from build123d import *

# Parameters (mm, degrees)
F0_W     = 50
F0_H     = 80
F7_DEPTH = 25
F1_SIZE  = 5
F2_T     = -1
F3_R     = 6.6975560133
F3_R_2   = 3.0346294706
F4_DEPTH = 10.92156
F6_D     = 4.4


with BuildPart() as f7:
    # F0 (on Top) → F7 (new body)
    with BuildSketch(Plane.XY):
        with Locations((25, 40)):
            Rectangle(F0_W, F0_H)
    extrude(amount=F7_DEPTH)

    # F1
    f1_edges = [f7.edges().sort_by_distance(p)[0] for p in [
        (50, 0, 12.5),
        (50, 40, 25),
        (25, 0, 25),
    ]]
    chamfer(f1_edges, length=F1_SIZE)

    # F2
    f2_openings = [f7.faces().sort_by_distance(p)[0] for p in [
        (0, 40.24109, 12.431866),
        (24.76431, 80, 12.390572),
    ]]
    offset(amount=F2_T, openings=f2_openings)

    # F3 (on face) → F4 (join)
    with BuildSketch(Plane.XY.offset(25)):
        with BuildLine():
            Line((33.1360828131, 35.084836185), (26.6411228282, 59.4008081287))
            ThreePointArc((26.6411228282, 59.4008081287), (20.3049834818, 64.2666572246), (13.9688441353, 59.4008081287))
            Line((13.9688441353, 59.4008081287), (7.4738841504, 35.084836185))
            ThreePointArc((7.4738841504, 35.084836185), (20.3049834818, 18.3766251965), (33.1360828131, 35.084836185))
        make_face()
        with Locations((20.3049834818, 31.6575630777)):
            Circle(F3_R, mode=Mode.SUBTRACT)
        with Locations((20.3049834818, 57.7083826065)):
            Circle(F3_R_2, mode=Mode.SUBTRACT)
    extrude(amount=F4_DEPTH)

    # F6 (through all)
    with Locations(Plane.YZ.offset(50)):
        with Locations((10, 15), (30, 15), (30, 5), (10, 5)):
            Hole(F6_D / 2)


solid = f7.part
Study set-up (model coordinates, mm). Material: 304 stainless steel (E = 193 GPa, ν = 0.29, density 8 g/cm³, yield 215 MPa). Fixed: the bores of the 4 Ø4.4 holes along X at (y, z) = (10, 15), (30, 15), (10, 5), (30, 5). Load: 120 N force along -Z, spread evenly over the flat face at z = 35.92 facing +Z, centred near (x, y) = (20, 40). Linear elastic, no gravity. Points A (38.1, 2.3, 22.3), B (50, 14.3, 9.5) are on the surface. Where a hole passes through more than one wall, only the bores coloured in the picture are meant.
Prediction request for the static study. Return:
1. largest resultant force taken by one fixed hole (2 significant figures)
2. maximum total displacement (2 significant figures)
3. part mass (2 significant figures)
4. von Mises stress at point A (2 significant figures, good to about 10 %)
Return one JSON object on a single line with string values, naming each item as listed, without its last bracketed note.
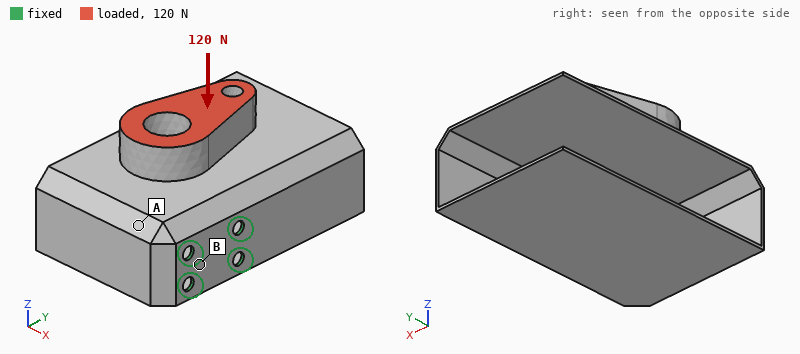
{"largest resultant force taken by one fixed hole": "240 N", "maximum total displacement": "0.60 mm", "part mass": "150 g", "von Mises stress at point A": "24 MPa"}
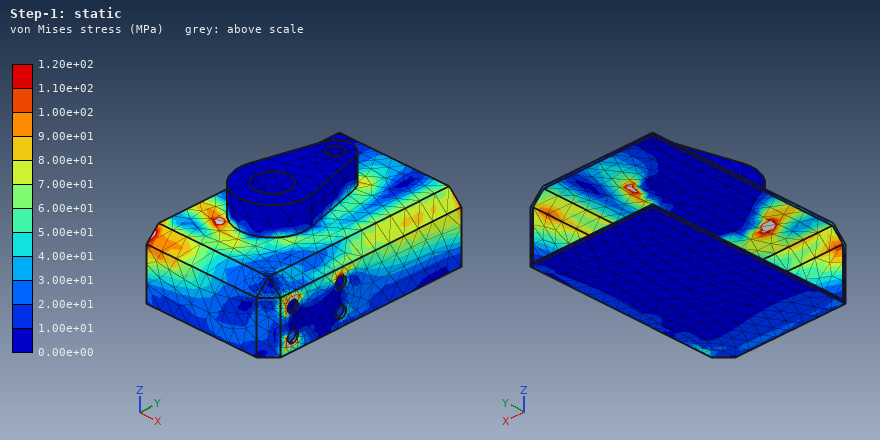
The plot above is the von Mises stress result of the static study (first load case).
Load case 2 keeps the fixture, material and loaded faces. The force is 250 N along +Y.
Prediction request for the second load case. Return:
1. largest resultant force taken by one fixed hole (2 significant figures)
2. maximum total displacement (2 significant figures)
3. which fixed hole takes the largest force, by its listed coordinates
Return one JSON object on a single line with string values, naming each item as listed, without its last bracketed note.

{"largest resultant force taken by one fixed hole": "380 N", "maximum total displacement": "0.34 mm", "which fixed hole takes the largest force, by its listed coordinates": "(10, 15)"}
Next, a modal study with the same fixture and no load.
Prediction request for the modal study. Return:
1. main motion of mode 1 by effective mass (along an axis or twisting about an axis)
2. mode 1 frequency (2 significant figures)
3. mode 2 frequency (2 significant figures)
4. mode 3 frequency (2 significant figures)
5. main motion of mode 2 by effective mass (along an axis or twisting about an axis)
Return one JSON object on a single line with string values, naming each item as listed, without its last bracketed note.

{"main motion of mode 1 by effective mass": "along Z", "mode 1 frequency": "330 Hz", "mode 2 frequency": "390 Hz", "mode 3 frequency": "660 Hz", "main motion of mode 2 by effective mass": "along Z"}
